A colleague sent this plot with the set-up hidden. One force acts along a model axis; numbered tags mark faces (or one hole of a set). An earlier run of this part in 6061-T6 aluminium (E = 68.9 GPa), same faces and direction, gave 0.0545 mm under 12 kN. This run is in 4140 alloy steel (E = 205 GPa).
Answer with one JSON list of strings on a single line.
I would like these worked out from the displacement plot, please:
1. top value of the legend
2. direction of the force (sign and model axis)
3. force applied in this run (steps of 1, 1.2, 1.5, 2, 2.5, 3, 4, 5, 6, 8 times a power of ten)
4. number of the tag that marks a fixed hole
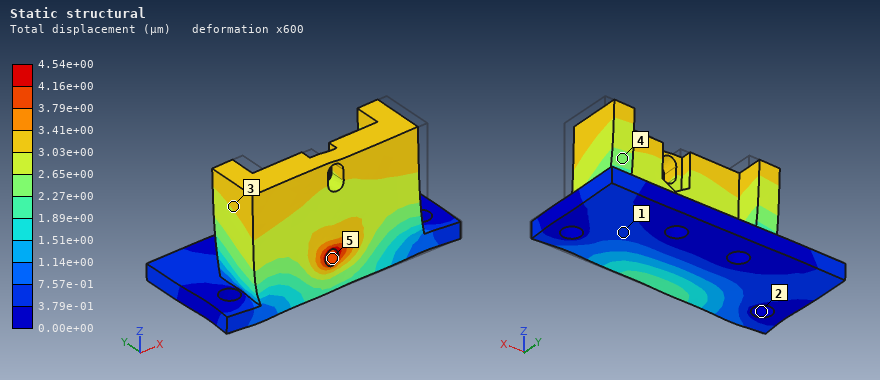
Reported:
["4.54e+00 µm", "-X", "3 kN", "2"]
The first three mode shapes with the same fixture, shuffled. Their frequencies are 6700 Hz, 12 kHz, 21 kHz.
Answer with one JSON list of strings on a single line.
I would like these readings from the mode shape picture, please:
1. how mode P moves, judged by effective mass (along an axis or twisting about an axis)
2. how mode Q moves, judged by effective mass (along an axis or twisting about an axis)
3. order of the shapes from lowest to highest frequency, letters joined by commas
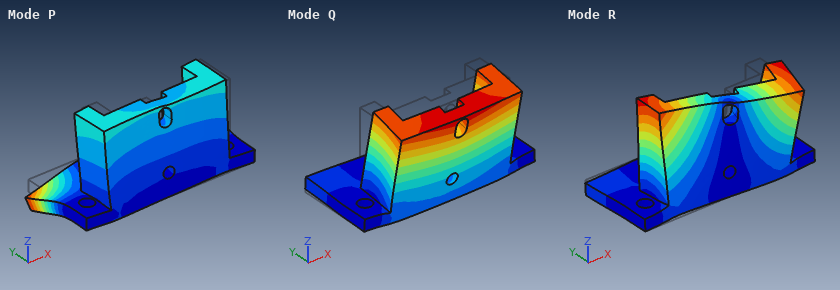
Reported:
["along X", "along Y", "Q, R, P"]
